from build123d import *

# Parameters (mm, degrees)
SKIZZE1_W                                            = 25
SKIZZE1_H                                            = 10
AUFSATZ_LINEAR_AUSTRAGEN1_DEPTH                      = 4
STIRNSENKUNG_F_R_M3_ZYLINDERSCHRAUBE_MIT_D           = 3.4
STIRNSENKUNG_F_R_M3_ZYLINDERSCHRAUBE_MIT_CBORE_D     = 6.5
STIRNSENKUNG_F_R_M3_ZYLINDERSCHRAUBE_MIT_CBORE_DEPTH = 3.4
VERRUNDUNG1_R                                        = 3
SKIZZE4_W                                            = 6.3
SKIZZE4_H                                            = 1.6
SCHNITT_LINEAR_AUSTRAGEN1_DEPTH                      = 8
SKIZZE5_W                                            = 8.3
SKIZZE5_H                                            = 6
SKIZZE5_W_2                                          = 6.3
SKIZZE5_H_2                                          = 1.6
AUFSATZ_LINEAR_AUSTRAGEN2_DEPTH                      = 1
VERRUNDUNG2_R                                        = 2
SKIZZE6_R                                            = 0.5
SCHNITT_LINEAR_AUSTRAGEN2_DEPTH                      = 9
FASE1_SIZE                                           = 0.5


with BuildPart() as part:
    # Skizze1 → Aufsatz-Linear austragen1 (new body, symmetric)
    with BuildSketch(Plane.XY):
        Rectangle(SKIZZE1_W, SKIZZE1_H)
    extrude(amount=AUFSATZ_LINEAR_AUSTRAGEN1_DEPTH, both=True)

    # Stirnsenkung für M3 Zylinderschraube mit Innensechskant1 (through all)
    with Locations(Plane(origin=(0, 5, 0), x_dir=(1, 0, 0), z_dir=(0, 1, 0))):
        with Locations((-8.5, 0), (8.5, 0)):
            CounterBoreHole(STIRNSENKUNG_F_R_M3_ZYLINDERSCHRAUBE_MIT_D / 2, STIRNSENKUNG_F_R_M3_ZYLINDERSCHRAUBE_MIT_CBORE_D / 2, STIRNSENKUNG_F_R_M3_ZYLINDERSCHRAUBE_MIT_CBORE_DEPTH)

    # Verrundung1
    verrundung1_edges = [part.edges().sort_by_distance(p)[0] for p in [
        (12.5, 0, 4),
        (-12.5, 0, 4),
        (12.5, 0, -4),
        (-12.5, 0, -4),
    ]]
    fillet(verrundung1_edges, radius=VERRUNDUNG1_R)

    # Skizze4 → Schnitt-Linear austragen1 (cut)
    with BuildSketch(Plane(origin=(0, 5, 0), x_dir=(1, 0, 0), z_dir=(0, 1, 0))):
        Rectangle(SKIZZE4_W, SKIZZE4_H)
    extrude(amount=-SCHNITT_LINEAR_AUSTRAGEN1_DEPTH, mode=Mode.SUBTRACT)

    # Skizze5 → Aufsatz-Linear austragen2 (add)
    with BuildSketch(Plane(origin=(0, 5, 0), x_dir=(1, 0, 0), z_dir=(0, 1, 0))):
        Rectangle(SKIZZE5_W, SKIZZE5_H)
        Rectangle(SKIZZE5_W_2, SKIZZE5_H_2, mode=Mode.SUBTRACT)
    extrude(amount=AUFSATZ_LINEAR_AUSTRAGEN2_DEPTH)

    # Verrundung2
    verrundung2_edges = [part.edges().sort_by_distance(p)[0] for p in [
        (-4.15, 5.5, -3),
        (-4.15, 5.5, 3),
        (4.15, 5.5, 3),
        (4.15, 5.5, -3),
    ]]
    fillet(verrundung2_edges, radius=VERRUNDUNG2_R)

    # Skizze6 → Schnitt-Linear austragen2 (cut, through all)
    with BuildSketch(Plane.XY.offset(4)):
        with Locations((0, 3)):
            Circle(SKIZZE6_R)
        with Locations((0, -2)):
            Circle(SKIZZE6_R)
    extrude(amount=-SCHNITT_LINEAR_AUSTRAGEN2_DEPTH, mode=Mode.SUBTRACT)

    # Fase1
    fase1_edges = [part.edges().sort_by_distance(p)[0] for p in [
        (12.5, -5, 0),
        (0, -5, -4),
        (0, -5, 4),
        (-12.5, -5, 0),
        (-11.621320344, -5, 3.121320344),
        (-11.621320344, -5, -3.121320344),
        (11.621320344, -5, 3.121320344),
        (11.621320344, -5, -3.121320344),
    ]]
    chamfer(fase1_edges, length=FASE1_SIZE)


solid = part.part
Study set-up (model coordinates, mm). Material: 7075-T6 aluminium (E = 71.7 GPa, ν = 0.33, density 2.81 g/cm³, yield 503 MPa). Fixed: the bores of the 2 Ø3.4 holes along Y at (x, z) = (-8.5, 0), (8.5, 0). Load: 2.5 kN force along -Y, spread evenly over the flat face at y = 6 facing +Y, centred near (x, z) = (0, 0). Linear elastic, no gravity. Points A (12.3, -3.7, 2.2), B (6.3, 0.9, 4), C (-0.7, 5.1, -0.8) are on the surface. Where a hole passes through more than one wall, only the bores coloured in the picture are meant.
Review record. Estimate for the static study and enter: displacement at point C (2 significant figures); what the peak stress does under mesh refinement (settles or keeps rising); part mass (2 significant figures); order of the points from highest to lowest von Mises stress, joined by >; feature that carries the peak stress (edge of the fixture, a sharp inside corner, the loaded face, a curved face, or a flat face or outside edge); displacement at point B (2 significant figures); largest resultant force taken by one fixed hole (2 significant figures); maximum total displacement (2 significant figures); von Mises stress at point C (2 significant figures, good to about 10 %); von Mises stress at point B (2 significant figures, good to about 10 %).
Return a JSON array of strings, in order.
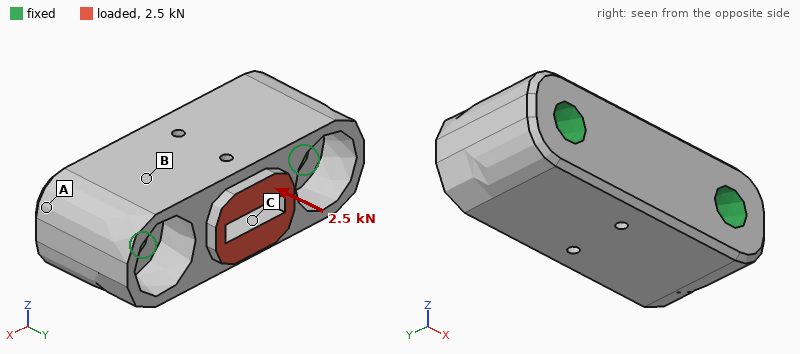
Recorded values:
["9.0 µm", "keeps rising", "4.3 g", "C > B > A", "a sharp inside corner", "2.4 µm", "1.3 kN", "10.0 µm", "60 MPa", "30 MPa"]
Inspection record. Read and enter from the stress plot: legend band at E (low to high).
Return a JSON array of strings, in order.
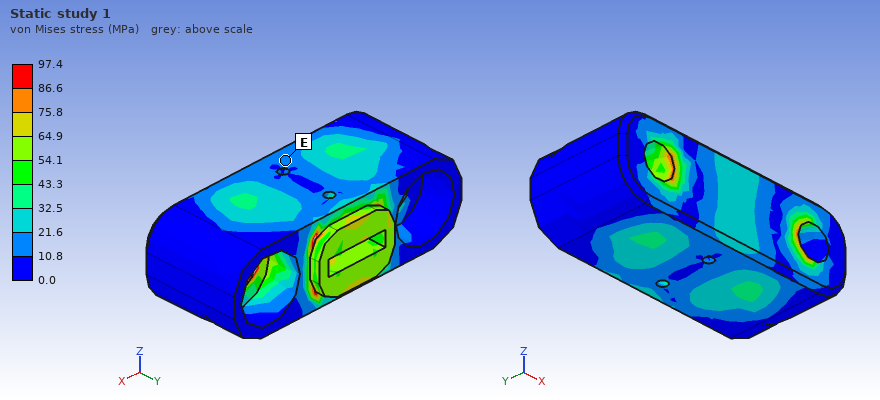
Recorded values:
["10.8 to 21.6 MPa"]
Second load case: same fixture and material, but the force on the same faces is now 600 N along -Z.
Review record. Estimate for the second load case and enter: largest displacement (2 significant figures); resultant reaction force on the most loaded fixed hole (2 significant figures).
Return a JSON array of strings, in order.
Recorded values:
["14 µm", "300 N"]
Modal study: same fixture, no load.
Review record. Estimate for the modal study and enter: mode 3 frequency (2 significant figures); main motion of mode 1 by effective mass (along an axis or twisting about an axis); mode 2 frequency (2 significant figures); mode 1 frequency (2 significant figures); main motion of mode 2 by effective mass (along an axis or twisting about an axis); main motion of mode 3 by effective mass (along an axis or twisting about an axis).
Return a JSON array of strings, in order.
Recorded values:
["81 kHz", "along Z", "76 kHz", "52 kHz", "along Y", "along Z"]
